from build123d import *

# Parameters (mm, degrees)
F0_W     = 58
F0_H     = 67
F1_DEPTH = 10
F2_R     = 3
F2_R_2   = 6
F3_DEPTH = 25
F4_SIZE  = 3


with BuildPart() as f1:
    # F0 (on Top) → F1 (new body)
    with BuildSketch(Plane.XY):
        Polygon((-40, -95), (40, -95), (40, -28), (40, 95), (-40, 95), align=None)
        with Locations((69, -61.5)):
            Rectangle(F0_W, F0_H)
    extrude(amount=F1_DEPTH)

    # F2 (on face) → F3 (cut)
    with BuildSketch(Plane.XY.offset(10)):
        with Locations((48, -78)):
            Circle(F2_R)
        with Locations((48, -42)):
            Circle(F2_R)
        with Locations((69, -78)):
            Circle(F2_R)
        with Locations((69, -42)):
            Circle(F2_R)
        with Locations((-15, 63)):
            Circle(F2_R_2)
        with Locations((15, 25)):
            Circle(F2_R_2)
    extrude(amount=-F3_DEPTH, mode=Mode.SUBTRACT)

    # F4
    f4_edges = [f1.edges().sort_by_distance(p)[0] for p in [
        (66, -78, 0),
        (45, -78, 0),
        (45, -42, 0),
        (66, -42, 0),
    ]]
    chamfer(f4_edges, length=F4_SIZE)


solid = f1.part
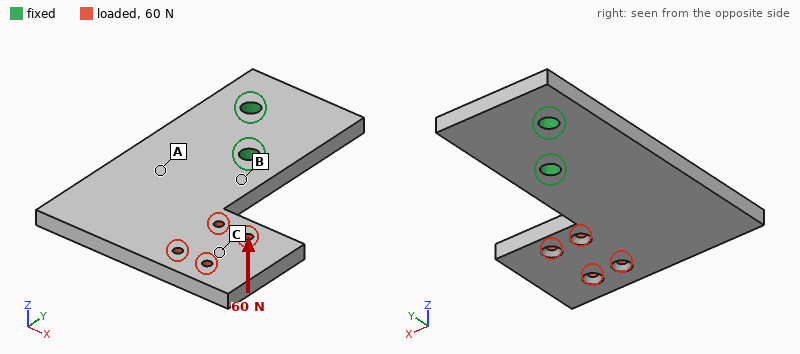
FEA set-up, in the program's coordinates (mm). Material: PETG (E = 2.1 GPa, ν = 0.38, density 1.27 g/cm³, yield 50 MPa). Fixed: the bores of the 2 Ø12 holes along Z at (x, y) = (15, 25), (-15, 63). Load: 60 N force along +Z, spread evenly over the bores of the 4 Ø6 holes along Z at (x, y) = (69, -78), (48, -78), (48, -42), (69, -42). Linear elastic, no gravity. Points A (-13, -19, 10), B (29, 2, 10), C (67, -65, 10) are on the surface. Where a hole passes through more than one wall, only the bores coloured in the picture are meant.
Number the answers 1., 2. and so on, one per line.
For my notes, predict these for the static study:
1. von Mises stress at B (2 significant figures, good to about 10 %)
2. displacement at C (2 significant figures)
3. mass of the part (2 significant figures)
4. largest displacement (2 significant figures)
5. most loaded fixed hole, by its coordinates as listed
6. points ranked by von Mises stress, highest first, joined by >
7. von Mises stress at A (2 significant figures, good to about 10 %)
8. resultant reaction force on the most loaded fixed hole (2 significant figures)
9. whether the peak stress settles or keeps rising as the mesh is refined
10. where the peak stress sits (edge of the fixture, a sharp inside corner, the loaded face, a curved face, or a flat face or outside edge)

1. 3.7 MPa
2. 1.7 mm
3. 240 g
4. 2.6 mm
5. (15, 25)
6. B > A > C
7. 2.3 MPa
8. 110 N
9. keeps rising
10. edge of the fixture
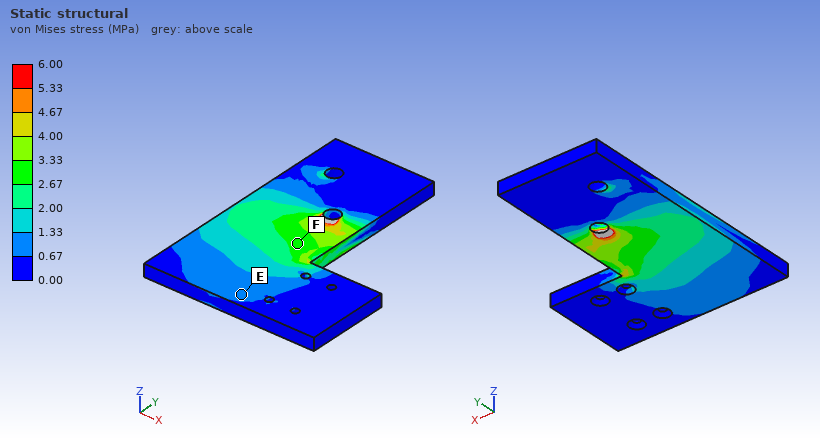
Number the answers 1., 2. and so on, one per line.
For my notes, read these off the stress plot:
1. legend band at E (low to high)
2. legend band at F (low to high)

1. 0.67 to 1.33 MPa
2. 2.67 to 3.33 MPa
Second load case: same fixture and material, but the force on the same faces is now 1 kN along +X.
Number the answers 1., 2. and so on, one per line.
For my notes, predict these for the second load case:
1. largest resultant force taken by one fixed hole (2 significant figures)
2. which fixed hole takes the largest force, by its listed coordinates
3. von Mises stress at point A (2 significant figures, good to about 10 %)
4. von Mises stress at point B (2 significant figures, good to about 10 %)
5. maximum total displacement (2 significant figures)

1. 2.2 kN
2. (15, 25)
3. 3.8 MPa
4. 4.4 MPa
5. 1.5 mm
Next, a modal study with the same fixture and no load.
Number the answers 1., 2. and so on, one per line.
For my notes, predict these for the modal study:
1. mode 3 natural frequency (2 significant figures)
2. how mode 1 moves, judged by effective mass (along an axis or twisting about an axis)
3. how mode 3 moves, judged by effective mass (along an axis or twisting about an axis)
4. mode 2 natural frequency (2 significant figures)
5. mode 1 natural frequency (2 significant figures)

1. 480 Hz
2. along Z
3. along X
4. 180 Hz
5. 110 Hz
